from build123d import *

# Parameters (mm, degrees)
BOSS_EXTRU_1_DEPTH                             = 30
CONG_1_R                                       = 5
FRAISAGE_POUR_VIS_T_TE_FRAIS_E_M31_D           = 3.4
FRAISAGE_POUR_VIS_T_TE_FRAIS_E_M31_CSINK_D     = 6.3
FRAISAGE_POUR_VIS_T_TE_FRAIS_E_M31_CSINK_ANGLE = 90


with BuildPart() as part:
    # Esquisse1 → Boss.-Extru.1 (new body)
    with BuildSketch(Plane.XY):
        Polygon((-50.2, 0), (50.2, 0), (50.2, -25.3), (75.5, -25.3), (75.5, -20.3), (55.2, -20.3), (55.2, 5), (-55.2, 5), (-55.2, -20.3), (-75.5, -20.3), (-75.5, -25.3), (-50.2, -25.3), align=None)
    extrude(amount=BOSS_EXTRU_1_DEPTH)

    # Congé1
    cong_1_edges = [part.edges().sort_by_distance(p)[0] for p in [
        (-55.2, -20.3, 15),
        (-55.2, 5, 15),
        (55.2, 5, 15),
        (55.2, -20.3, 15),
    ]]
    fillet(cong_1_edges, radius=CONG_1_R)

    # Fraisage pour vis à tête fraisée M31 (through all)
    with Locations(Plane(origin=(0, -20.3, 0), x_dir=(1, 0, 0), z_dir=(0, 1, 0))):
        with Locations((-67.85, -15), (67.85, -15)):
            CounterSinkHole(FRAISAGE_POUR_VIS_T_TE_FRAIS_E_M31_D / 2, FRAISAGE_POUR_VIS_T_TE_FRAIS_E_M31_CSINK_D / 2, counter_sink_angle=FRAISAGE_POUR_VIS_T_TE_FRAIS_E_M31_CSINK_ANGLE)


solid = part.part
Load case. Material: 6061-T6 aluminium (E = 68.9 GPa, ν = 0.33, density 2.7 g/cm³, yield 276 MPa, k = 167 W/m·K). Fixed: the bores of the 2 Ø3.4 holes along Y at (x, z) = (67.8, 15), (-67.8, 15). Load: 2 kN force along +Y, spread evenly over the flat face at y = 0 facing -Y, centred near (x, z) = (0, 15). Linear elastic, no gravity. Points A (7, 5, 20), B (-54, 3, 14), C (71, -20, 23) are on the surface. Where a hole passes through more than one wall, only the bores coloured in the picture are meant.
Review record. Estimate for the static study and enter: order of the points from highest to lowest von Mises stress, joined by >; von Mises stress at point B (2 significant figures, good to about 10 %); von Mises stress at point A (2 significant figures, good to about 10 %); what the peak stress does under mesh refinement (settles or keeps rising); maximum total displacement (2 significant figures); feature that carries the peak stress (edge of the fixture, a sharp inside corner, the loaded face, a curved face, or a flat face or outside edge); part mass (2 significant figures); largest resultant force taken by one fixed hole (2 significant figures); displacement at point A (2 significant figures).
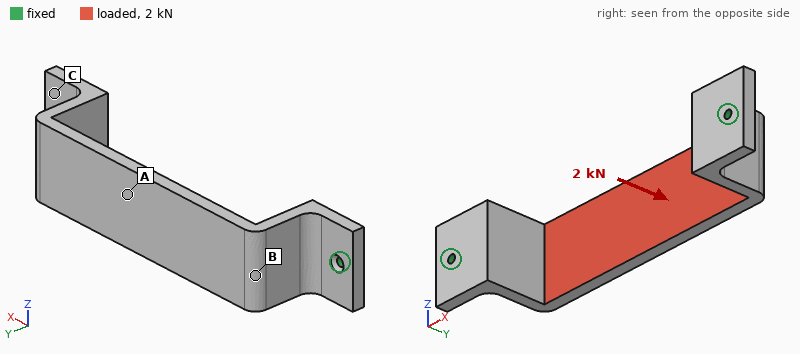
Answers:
A > B > C
53 MPa
85 MPa
keeps rising
0.41 mm
edge of the fixture
81 g
1.5 kN
0.39 mm
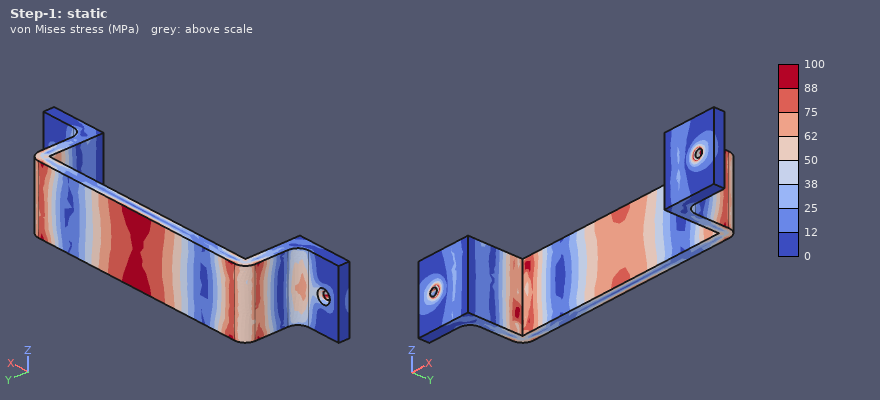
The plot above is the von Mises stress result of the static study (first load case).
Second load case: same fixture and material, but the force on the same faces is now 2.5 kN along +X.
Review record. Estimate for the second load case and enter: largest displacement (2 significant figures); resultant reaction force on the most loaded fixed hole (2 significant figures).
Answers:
0.39 mm
1.3 kN
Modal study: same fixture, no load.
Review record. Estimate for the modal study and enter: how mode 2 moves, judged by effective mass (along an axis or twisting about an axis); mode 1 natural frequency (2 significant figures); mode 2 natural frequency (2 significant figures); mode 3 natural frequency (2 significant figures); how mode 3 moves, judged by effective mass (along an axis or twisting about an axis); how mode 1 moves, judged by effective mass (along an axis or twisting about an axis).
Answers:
along X
1400 Hz
1800 Hz
2000 Hz
along Y
along Z
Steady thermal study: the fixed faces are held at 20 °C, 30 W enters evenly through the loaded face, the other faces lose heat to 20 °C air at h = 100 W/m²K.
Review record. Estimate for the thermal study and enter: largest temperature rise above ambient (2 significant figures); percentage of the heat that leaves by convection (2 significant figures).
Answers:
25 K
46 %
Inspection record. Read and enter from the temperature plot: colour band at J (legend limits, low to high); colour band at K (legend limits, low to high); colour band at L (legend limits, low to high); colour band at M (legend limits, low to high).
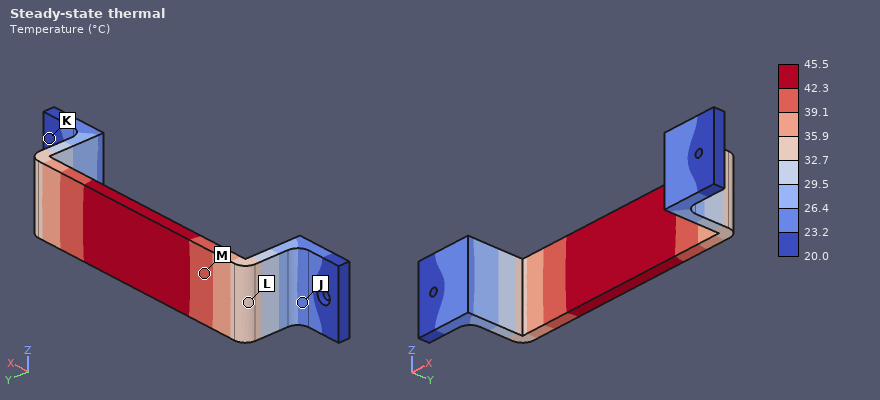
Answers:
23.2 to 26.4 °C
20.0 to 23.2 °C
32.7 to 35.9 °C
39.1 to 42.3 °C
